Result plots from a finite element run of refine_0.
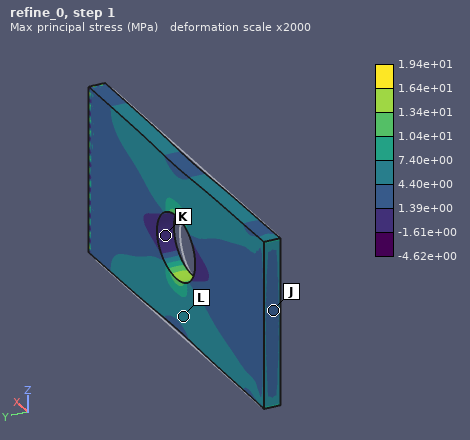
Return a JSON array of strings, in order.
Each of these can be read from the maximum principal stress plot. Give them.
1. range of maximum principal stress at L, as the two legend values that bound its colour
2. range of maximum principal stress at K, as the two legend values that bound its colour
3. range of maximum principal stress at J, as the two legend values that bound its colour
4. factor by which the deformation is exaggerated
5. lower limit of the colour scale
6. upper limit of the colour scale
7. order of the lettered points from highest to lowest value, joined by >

["4.40e+00 to 7.40e+00 MPa", "-1.61e+00 to 1.39e+00 MPa", "1.39e+00 to 4.40e+00 MPa", "2000", "-4.62e+00 MPa", "1.94e+01 MPa", "L > J > K"]
